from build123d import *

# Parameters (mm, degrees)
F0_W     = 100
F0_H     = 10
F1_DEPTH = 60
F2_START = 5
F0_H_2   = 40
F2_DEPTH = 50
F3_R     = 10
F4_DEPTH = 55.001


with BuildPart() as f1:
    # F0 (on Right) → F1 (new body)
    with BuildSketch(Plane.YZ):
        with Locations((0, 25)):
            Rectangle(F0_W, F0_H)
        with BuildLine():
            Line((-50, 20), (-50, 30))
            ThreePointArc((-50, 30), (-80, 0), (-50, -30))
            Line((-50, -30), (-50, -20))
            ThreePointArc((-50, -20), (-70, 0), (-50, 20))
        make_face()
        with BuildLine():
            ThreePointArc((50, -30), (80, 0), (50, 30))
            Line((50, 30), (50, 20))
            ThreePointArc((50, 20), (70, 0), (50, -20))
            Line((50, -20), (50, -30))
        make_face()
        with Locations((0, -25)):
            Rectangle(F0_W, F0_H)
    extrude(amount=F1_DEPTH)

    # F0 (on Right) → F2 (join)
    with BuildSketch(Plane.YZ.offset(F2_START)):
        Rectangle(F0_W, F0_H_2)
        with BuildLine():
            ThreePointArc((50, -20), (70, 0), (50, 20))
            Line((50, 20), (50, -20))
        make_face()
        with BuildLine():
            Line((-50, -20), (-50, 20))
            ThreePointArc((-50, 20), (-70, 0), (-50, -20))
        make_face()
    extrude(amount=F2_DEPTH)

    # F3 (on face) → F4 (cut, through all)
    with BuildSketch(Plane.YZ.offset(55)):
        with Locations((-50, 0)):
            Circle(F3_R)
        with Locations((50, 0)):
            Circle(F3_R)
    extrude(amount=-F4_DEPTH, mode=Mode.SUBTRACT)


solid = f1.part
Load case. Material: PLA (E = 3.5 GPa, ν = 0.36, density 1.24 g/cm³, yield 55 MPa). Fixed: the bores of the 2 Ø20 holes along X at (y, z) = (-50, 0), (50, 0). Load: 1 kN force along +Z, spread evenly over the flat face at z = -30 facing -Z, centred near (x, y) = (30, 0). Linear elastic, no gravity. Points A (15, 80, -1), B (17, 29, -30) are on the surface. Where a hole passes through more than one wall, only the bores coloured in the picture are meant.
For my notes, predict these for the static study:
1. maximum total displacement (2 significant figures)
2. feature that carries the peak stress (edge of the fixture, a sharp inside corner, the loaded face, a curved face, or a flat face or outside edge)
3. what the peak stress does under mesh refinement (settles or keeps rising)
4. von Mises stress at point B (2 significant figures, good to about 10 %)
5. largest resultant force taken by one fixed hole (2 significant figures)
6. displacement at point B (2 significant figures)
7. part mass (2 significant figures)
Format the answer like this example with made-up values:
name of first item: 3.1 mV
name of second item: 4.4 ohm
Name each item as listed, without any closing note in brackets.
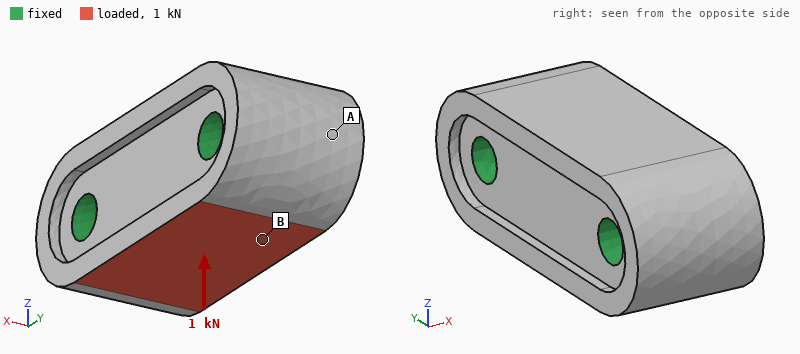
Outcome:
maximum total displacement: 6.9 µm
feature that carries the peak stress: edge of the fixture
what the peak stress does under mesh refinement: keeps rising
von Mises stress at point B: 0.24 MPa
largest resultant force taken by one fixed hole: 510 N
displacement at point B: 3.6 µm
part mass: 550 g
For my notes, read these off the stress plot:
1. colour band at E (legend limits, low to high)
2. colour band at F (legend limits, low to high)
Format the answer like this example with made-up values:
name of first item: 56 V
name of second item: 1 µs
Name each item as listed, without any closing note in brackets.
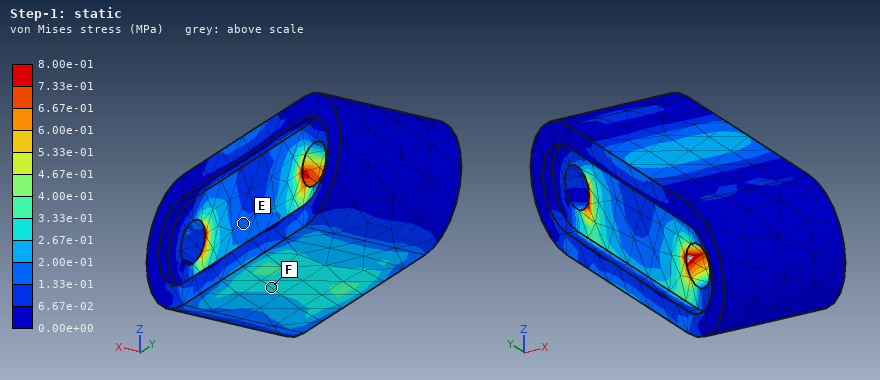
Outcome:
colour band at E: 1.33e-01 to 2.00e-01 MPa
colour band at F: 2.67e-01 to 3.33e-01 MPa
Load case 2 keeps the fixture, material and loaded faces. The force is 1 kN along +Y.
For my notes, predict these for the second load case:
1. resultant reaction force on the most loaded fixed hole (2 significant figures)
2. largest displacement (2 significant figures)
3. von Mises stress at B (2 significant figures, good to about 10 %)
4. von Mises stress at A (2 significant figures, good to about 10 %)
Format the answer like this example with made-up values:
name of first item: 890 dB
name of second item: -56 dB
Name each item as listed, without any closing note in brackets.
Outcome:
resultant reaction force on the most loaded fixed hole: 550 N
largest displacement: 4.1 µm
von Mises stress at B: 0.30 MPa
von Mises stress at A: 0.069 MPa
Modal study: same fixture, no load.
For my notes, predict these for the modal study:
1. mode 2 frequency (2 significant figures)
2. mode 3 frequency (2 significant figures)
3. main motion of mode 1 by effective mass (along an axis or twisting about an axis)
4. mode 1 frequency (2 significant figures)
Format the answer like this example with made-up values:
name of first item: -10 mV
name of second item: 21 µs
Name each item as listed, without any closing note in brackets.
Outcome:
mode 2 frequency: 4300 Hz
mode 3 frequency: 4400 Hz
main motion of mode 1 by effective mass: along Z
mode 1 frequency: 4100 Hz
